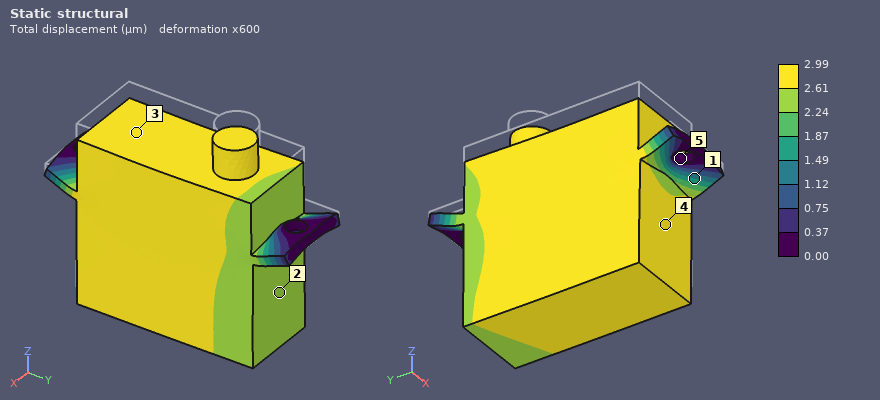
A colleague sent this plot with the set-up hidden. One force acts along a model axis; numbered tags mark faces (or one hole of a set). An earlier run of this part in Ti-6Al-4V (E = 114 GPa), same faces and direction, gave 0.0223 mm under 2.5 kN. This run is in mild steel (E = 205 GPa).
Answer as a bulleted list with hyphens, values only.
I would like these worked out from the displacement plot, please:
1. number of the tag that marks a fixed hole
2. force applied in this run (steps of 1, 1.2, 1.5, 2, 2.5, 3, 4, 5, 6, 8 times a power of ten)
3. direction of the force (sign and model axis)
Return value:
- 5
- 600 N
- -Z
